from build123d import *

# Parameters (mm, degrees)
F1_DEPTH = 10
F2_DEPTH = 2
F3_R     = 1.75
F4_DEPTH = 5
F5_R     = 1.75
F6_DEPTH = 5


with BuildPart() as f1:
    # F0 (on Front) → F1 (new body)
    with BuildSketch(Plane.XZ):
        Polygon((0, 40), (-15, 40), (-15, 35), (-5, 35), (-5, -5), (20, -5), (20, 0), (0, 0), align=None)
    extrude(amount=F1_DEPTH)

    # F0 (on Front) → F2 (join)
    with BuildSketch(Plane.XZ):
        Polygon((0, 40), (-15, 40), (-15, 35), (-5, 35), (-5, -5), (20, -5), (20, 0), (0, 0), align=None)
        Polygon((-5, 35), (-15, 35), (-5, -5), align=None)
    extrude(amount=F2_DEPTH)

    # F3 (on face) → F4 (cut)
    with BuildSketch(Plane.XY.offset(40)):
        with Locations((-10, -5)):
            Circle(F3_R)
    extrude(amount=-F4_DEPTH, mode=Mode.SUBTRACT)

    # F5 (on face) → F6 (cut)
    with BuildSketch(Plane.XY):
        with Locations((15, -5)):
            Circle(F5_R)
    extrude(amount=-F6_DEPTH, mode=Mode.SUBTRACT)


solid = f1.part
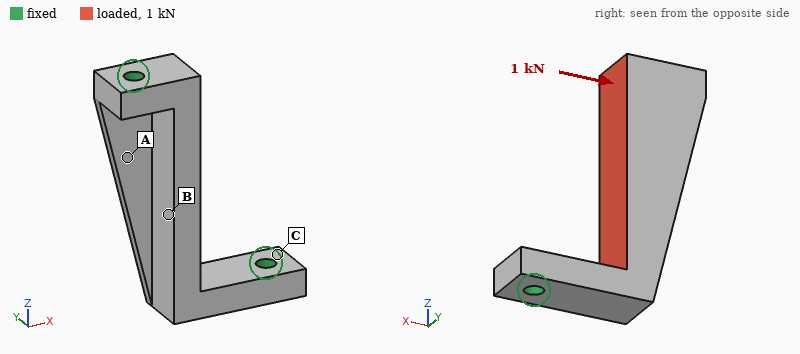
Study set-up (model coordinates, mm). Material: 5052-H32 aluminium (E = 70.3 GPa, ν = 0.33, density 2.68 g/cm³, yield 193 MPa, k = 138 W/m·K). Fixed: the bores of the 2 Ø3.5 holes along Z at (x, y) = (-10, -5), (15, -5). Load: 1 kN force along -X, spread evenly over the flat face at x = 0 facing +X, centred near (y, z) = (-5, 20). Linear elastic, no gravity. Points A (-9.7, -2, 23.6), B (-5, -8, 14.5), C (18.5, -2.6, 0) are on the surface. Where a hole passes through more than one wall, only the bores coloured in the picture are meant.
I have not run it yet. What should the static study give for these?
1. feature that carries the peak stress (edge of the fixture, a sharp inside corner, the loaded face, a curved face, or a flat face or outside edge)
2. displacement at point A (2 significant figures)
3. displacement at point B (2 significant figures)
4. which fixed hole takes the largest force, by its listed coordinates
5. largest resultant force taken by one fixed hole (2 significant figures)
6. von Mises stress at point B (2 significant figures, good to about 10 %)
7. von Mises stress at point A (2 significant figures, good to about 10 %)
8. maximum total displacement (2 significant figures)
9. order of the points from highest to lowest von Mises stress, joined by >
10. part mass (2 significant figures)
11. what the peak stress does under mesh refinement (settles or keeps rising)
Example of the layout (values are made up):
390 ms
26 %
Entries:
edge of the fixture
18 µm
30 µm
(-10, -5)
590 N
36 MPa
21 MPa
33 µm
B > A > C
11 g
keeps rising
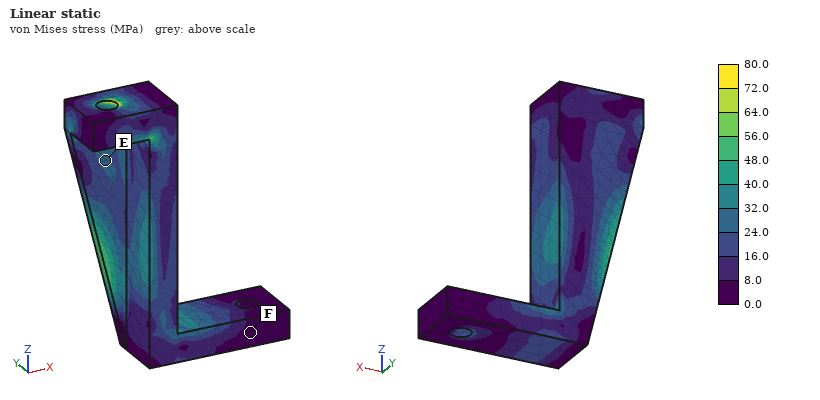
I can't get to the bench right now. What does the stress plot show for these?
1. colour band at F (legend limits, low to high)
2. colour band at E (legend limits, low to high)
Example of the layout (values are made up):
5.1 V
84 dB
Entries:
0.0 to 8.0 MPa
24.0 to 32.0 MPa
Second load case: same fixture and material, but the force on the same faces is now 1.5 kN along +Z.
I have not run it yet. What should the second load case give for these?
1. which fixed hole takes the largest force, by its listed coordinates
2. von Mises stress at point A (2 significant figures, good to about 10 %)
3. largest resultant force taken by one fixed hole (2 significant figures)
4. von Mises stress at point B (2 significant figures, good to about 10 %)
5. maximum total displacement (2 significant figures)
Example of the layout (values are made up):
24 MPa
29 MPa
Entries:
(-10, -5)
36 MPa
1.4 kN
22 MPa
26 µm
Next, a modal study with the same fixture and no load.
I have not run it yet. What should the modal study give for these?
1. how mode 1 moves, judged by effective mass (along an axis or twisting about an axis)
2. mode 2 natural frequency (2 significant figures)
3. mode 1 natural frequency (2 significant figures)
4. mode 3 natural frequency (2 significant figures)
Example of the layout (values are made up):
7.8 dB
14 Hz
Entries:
along Y
12 kHz
8800 Hz
18 kHz
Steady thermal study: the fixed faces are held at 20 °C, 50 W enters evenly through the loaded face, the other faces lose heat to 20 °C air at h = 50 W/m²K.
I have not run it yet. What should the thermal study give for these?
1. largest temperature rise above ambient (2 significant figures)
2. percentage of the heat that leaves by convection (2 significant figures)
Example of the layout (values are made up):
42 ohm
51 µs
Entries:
55 K
6.2 %
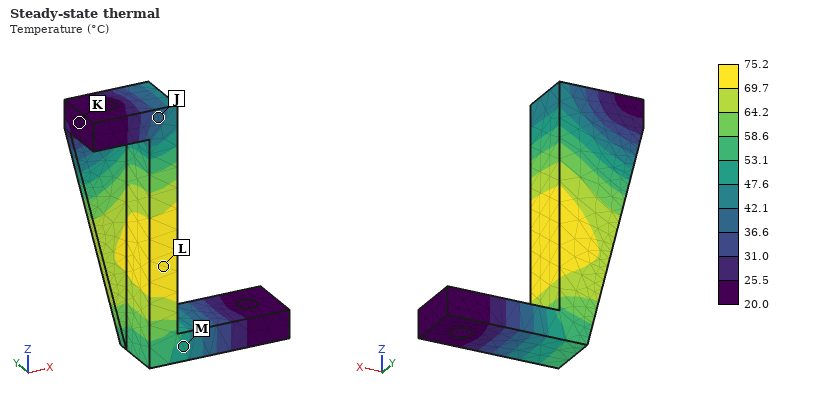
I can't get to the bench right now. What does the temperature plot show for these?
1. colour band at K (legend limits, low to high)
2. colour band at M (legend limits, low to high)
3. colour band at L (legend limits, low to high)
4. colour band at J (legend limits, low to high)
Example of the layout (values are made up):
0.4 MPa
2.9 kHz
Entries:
20.0 to 25.5 °C
47.6 to 53.1 °C
69.7 to 75.2 °C
36.6 to 42.1 °C
